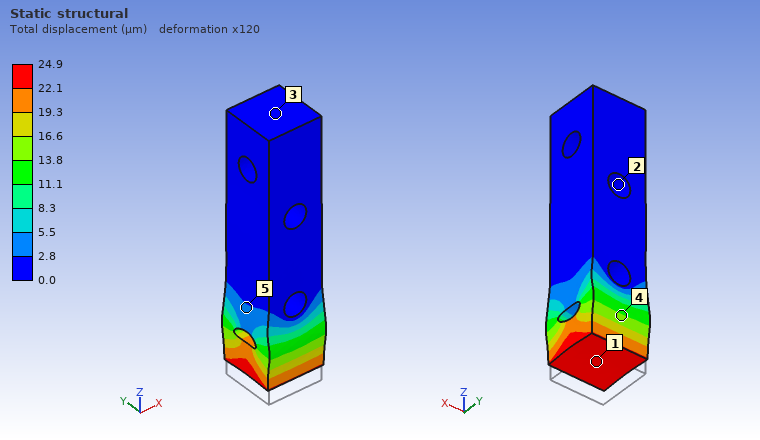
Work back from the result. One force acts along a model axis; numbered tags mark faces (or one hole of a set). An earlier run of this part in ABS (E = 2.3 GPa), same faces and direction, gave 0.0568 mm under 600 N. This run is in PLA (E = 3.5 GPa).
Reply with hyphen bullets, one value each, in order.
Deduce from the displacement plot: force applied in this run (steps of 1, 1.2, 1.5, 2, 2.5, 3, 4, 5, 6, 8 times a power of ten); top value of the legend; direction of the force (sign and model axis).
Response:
- 400 N
- 24.9 µm
- +Z
